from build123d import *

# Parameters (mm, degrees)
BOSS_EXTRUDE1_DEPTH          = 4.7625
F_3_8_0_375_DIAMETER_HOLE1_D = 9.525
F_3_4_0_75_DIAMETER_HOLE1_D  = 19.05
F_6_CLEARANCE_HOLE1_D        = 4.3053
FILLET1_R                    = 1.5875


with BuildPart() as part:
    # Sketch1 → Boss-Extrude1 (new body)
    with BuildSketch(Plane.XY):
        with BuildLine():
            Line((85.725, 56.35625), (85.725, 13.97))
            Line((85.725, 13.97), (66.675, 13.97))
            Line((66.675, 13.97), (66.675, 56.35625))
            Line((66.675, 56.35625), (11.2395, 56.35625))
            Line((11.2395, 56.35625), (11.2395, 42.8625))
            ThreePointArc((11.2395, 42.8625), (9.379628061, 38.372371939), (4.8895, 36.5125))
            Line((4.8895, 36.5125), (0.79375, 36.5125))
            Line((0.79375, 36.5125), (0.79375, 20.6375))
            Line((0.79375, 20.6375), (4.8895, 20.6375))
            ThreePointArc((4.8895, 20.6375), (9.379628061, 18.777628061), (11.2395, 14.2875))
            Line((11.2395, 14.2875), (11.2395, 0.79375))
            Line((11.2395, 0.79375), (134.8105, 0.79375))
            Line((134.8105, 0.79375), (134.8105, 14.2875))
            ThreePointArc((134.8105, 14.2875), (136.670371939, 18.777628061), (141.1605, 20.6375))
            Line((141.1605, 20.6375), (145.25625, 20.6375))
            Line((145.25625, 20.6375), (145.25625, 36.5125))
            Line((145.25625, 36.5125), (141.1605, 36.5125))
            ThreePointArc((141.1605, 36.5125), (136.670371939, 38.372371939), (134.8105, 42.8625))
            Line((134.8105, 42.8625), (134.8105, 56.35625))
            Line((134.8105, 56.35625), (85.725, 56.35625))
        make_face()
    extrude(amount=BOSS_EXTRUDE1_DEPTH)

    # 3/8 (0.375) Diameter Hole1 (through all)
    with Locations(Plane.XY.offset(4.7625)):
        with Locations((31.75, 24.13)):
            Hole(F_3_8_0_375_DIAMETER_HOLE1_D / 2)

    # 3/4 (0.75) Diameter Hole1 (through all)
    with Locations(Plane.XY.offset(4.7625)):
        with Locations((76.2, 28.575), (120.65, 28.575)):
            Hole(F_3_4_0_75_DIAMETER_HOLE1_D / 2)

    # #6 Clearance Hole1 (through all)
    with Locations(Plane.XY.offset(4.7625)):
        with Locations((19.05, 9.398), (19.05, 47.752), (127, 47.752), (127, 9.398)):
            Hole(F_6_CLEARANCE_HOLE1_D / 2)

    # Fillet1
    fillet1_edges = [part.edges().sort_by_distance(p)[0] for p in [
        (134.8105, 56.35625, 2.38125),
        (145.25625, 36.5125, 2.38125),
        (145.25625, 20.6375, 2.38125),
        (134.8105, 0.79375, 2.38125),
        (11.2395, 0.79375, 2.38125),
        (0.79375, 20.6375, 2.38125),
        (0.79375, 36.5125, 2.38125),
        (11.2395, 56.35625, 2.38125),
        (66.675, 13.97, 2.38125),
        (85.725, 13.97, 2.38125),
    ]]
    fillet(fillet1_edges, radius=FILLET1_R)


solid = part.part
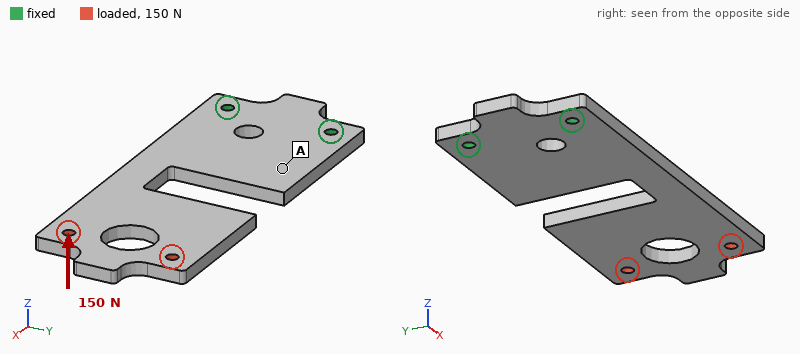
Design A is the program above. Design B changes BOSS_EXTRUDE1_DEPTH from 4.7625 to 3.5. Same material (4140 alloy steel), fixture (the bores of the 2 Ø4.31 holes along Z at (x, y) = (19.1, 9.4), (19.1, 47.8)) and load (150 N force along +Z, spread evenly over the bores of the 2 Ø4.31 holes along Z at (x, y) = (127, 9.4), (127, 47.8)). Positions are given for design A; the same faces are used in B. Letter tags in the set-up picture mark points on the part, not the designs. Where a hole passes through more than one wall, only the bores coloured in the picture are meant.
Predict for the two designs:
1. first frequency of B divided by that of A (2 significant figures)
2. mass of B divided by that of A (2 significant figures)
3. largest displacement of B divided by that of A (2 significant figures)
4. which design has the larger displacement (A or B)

0.74
0.73
2.5
B
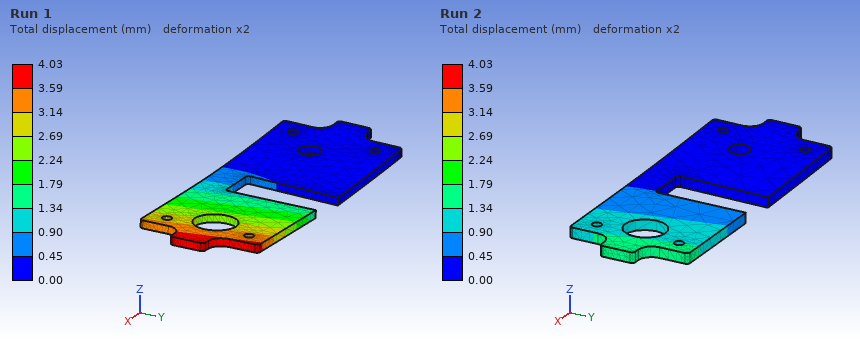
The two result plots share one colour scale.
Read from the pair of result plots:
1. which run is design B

Run 1
